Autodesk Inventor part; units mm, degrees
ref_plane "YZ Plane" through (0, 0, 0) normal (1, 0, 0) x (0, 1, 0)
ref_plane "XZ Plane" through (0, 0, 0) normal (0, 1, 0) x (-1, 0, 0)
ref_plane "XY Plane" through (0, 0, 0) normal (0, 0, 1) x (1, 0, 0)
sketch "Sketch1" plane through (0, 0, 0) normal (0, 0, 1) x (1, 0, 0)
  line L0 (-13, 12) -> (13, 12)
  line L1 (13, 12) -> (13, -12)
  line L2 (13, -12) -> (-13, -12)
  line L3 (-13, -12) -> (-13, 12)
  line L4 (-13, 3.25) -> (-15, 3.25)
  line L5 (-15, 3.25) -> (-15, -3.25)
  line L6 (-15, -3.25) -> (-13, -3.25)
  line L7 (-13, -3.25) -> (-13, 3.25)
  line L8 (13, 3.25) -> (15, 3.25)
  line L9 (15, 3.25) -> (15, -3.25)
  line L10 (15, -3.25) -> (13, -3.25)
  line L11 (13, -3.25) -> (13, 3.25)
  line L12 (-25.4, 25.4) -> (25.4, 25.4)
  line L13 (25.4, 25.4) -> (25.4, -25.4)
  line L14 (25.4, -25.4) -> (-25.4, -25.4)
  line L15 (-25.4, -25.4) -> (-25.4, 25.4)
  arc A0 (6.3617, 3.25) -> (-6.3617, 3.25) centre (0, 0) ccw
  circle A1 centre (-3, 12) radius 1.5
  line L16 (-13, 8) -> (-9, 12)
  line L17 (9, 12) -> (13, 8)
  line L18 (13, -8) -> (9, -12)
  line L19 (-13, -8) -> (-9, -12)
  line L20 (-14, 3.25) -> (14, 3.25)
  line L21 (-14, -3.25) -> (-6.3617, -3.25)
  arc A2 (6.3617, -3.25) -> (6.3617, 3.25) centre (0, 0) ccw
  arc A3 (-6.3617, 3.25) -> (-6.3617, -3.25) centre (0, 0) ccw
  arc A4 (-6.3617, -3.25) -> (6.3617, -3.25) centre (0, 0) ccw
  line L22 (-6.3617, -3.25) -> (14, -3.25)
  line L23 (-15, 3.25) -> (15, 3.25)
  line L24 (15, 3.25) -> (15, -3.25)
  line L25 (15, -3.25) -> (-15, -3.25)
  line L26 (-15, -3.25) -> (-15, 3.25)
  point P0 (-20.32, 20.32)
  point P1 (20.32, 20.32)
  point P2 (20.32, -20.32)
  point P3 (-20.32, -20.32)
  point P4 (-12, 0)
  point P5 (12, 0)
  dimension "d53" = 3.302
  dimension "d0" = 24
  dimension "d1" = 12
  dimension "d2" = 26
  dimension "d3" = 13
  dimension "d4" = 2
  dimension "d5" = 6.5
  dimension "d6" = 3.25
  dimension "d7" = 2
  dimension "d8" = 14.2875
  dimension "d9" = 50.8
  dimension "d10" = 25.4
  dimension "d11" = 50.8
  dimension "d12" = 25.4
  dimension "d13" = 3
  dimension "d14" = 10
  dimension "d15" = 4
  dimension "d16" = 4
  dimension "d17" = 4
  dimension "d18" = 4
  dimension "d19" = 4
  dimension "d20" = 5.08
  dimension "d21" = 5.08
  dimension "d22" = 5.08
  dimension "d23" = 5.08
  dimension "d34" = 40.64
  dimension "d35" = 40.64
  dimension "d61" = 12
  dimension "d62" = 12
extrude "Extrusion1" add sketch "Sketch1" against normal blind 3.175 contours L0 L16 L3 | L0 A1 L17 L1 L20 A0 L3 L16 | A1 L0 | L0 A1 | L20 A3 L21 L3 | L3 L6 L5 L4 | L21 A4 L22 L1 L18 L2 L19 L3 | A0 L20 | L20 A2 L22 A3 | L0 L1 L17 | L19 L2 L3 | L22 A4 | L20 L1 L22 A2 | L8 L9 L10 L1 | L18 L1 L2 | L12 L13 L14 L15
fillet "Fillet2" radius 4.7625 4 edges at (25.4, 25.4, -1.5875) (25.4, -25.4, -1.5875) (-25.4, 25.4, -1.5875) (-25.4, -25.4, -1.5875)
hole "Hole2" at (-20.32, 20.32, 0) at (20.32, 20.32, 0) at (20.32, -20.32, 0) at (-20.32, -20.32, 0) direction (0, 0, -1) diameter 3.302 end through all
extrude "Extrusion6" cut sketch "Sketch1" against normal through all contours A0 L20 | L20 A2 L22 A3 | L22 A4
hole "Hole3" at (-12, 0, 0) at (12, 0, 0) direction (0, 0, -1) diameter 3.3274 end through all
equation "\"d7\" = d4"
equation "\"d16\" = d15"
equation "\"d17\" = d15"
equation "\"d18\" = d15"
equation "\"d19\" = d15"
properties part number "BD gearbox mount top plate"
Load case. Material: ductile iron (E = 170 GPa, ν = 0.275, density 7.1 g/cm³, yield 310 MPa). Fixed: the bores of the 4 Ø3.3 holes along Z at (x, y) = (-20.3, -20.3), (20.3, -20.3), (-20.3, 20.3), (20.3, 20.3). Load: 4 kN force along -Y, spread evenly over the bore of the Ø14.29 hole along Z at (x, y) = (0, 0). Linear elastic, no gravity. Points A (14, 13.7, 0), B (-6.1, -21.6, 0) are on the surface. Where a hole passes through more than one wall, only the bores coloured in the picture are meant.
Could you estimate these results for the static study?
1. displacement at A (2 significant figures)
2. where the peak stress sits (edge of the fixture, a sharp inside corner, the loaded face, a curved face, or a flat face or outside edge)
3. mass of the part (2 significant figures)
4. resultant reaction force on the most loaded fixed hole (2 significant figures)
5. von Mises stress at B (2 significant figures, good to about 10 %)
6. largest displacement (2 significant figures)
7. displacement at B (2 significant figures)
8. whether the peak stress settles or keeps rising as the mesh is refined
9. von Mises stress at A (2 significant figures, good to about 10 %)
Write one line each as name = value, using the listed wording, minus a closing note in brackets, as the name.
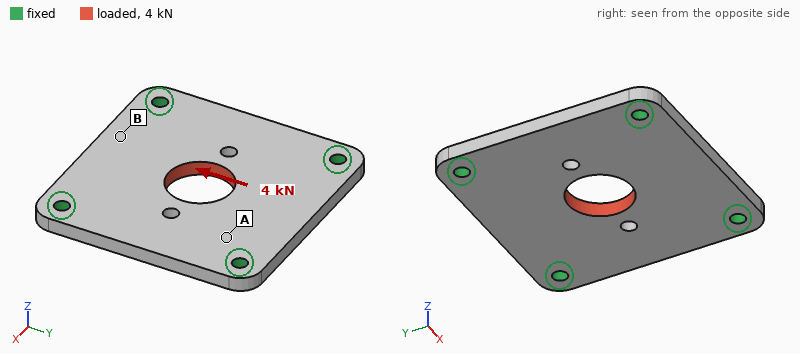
displacement at A = 2.1 µm
where the peak stress sits = edge of the fixture
mass of the part = 53 g
resultant reaction force on the most loaded fixed hole = 1.1 kN
von Mises stress at B = 11 MPa
largest displacement = 5.4 µm
displacement at B = 3.7 µm
whether the peak stress settles or keeps rising as the mesh is refined = keeps rising
von Mises stress at A = 29 MPa
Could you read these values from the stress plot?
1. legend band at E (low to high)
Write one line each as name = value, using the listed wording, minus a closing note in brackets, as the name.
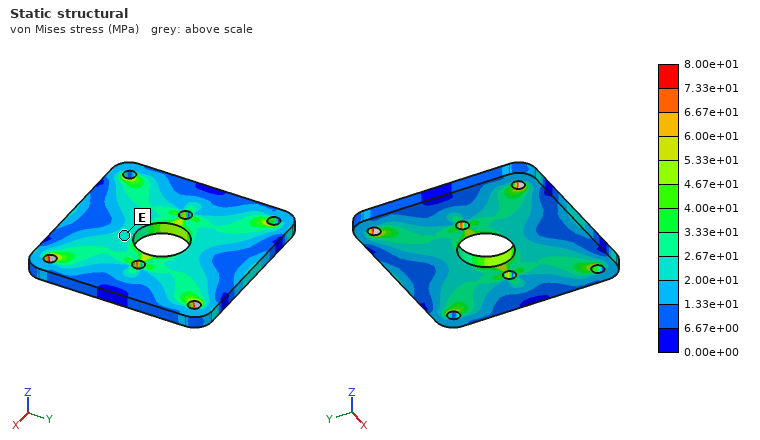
legend band at E = 2.00e+01 to 2.67e+01 MPa
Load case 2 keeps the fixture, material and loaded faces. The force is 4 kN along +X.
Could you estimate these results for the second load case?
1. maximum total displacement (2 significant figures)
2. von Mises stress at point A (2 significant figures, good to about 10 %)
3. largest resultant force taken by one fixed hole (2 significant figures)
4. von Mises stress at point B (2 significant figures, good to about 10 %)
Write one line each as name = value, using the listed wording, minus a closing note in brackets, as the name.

maximum total displacement = 5.5 µm
von Mises stress at point A = 29 MPa
largest resultant force taken by one fixed hole = 1.1 kN
von Mises stress at point B = 10 MPa
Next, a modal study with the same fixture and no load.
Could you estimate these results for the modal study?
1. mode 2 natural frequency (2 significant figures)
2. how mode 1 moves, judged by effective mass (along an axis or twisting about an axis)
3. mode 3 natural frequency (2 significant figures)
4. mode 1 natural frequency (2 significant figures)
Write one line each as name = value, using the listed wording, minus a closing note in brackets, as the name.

mode 2 natural frequency = 10 kHz
how mode 1 moves, judged by effective mass = along Z
mode 3 natural frequency = 10 kHz
mode 1 natural frequency = 6700 Hz
